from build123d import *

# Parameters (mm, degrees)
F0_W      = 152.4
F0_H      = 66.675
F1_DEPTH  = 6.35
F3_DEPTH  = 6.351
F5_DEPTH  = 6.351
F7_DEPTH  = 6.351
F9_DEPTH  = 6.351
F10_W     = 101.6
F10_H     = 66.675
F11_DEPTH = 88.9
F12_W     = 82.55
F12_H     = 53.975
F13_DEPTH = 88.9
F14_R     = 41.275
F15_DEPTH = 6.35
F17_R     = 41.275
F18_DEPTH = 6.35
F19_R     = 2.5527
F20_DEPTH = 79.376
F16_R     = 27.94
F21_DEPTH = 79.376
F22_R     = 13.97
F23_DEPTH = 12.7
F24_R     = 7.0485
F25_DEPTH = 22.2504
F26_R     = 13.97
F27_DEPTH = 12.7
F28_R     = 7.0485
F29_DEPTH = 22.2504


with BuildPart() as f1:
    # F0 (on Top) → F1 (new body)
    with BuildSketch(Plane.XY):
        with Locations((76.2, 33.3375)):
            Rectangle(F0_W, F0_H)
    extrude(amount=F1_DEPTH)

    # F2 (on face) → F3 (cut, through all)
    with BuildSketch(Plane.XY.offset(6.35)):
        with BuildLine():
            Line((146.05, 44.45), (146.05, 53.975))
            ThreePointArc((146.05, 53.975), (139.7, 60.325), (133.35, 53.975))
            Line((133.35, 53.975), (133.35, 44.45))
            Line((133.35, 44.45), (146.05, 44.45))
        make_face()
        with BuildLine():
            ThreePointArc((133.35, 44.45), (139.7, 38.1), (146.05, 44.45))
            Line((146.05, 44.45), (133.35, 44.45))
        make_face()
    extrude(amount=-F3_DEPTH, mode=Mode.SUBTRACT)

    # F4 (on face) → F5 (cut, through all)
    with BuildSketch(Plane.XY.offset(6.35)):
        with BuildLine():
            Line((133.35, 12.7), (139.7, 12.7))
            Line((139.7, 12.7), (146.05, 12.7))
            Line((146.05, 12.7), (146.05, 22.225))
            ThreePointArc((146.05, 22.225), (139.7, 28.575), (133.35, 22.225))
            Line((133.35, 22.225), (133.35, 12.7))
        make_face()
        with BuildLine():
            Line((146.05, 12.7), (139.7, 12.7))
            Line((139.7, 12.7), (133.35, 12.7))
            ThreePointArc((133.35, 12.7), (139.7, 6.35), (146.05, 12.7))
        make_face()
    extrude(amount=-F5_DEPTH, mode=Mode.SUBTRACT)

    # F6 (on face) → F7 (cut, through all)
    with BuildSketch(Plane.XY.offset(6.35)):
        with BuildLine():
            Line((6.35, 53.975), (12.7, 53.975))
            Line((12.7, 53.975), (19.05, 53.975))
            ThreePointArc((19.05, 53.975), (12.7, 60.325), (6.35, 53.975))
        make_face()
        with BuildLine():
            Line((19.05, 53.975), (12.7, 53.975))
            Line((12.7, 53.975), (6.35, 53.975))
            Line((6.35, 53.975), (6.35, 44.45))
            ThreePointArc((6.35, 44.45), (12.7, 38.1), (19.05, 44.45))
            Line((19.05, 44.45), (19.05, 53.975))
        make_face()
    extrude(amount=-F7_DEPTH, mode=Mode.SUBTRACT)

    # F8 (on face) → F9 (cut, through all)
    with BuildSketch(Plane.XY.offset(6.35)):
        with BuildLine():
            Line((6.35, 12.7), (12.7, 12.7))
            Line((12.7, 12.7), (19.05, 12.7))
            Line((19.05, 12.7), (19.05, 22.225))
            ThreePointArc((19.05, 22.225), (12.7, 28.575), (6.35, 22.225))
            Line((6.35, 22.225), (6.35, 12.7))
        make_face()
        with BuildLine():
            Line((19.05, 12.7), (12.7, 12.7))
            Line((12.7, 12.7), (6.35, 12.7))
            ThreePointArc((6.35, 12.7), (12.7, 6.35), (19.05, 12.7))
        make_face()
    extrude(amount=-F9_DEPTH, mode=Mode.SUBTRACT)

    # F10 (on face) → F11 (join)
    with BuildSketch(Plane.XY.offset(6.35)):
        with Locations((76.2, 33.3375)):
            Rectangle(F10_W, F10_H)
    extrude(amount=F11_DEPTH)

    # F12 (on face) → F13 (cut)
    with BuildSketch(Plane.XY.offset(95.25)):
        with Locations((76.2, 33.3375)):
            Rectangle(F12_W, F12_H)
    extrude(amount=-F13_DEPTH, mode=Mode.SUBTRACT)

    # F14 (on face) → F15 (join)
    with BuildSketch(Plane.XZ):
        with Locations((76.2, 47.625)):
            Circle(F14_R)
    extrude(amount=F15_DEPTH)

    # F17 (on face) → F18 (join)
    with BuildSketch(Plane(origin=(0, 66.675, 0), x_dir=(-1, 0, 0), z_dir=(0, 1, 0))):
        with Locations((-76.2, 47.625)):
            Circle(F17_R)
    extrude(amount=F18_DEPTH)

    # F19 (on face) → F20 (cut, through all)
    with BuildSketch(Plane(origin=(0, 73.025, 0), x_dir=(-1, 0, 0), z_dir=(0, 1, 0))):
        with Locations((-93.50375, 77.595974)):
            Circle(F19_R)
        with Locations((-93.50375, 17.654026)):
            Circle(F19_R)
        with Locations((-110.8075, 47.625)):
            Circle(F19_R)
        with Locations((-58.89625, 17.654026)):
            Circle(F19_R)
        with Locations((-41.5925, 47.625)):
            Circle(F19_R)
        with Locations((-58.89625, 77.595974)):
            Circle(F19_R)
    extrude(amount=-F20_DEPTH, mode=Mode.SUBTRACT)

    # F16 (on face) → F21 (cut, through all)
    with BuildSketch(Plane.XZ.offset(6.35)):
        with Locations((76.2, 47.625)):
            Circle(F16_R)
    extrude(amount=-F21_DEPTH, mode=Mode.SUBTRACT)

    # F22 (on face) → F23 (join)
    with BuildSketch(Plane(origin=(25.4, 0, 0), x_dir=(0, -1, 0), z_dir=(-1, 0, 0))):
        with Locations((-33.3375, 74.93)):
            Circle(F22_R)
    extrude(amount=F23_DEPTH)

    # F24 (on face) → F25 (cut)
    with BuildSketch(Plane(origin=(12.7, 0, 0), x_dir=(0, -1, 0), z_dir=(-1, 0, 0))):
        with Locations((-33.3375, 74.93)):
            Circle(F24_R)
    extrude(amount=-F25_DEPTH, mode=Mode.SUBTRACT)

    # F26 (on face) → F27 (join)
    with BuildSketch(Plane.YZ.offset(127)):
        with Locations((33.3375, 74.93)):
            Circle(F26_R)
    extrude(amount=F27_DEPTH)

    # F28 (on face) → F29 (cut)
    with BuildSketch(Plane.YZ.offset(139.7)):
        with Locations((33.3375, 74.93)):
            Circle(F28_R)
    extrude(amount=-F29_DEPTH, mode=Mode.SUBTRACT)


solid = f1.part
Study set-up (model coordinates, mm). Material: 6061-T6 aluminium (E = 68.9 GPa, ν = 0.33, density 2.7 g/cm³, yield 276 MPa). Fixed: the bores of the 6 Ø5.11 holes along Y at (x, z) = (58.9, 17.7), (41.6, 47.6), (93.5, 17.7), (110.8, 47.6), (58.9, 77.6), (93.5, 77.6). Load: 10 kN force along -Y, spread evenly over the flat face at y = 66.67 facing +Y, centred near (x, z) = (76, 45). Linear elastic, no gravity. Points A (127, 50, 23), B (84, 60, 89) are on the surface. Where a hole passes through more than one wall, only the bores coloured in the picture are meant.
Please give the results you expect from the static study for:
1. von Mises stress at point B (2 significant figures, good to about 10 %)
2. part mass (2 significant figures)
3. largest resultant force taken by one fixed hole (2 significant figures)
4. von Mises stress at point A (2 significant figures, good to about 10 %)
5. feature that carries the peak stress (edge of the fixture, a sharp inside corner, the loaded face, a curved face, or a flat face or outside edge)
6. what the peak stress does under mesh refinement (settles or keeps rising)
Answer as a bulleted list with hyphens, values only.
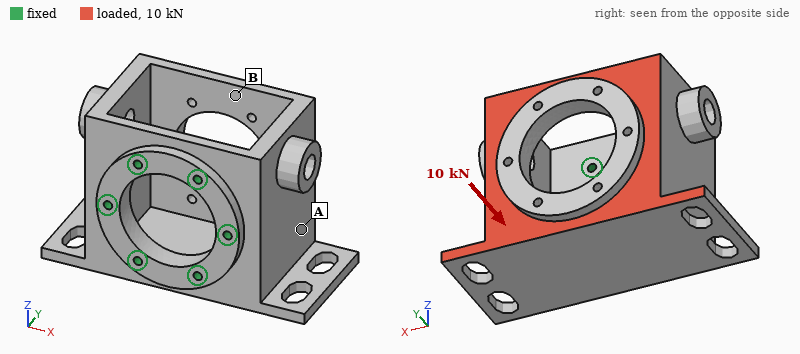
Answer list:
- 22 MPa
- 740 g
- 3.6 kN
- 7.2 MPa
- edge of the fixture
- keeps rising
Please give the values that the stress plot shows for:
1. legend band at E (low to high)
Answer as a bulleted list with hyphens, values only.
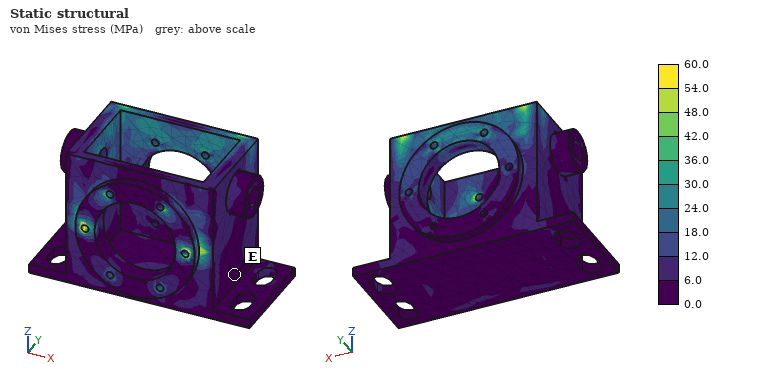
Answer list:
- 0.0 to 6.0 MPa
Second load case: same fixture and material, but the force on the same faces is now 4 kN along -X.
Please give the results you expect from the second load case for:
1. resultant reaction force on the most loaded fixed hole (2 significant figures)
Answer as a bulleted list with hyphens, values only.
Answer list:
- 2.8 kN
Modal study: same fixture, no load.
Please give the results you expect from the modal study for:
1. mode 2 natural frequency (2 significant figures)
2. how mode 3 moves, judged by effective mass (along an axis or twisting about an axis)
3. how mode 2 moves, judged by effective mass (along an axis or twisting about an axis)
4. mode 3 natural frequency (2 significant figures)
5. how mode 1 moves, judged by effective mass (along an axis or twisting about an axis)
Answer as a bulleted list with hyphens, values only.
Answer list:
- 2100 Hz
- along Y
- along Z
- 3900 Hz
- along X
